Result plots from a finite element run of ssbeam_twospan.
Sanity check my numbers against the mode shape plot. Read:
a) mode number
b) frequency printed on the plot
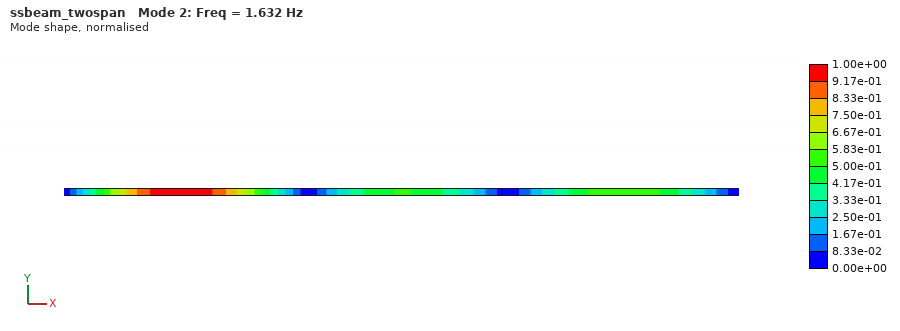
2
1.632 Hz
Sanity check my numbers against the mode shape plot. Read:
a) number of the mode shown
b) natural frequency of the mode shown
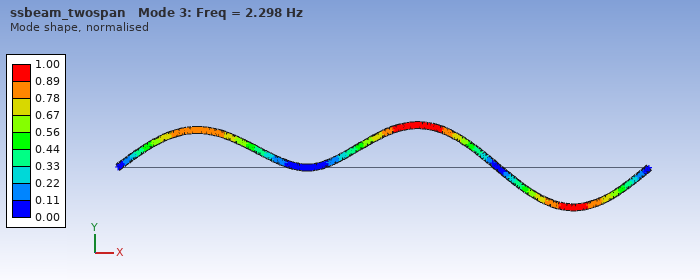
3
2.298 Hz
